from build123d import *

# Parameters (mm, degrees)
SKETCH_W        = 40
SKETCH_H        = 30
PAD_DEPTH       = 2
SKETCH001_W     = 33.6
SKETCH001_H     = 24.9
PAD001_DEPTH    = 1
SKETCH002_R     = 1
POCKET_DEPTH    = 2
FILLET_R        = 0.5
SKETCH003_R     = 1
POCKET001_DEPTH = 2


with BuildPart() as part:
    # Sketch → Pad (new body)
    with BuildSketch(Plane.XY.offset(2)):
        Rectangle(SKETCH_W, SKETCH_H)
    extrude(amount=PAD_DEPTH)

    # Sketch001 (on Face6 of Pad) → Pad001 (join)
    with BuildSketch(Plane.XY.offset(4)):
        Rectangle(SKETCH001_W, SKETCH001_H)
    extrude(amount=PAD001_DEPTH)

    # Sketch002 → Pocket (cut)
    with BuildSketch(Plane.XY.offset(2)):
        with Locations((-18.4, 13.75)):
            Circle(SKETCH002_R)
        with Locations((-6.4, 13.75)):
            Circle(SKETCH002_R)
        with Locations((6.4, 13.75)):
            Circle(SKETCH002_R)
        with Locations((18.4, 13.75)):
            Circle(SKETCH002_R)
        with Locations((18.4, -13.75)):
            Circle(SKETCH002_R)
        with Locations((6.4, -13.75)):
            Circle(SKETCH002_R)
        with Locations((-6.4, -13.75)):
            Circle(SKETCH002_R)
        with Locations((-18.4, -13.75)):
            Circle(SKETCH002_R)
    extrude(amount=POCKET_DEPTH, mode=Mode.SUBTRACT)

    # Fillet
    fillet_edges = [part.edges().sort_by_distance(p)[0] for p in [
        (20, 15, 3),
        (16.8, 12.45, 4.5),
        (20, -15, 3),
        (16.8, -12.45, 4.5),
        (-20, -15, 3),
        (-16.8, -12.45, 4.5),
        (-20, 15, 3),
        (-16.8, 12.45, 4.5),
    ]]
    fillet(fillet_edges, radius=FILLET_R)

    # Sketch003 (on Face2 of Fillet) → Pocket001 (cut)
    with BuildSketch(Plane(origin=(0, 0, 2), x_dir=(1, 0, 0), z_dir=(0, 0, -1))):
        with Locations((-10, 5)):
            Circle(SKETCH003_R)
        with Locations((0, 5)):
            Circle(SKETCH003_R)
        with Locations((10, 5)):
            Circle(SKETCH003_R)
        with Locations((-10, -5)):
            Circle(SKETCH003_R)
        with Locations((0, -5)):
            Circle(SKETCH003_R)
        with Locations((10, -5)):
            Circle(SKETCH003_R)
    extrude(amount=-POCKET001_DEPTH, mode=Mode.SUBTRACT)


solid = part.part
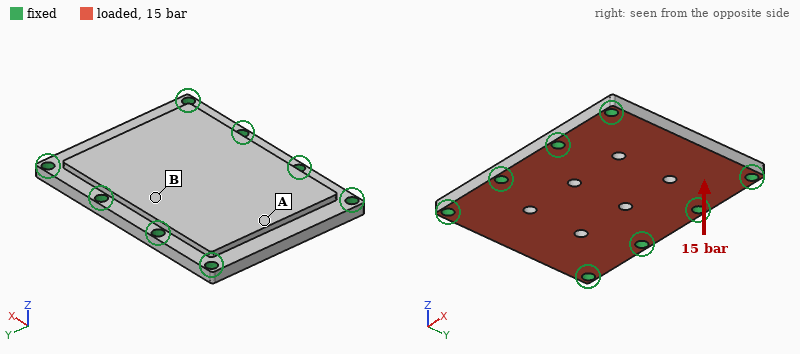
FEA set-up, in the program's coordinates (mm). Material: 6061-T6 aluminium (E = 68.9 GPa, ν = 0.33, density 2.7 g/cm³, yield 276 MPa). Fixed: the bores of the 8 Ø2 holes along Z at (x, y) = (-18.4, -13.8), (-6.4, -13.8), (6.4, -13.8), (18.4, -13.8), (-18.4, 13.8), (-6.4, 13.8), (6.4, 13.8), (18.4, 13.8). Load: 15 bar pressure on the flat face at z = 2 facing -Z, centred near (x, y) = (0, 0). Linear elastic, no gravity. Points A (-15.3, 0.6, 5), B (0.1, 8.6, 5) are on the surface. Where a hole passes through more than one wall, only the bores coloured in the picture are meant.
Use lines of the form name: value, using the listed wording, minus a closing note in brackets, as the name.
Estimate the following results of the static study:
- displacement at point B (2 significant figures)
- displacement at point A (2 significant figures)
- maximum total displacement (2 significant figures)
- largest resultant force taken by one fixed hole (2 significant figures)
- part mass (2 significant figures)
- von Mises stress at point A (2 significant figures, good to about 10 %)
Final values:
displacement at point B: 15 µm
displacement at point A: 32 µm
maximum total displacement: 37 µm
largest resultant force taken by one fixed hole: 320 N
part mass: 8.5 g
von Mises stress at point A: 58 MPa
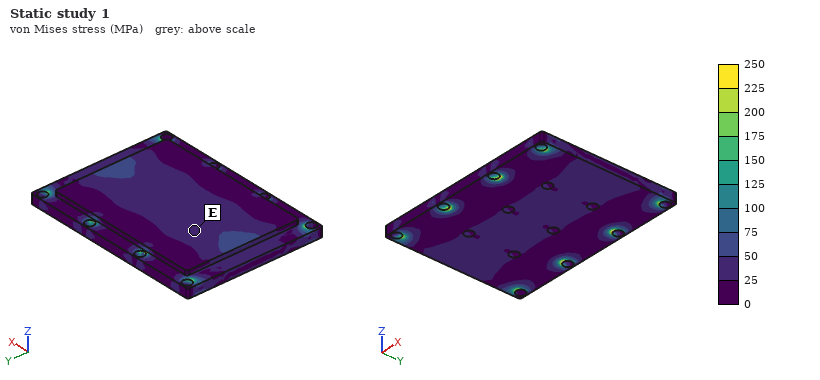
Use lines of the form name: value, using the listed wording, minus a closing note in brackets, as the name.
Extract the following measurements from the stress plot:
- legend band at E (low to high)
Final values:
legend band at E: 25 to 50 MPa
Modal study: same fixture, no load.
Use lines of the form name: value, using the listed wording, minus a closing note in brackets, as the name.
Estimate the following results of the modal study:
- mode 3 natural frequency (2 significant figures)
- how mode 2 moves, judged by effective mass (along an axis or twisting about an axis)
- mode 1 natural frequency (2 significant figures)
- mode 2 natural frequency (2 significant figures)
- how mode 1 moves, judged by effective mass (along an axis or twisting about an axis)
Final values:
mode 3 natural frequency: 24 kHz
how mode 2 moves, judged by effective mass: twisting about Y
mode 1 natural frequency: 14 kHz
mode 2 natural frequency: 17 kHz
how mode 1 moves, judged by effective mass: along Z
